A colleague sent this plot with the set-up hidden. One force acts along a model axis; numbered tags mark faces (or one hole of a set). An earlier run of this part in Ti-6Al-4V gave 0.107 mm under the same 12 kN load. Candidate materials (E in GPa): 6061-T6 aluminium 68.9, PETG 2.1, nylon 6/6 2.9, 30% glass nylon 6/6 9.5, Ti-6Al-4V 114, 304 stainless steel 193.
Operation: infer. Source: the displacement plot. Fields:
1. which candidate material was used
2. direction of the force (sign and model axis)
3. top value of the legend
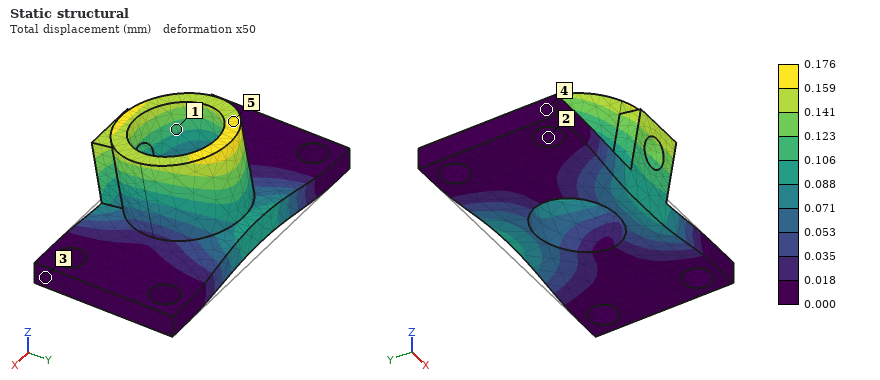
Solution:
6061-T6 aluminium
-Y
0.176 mm
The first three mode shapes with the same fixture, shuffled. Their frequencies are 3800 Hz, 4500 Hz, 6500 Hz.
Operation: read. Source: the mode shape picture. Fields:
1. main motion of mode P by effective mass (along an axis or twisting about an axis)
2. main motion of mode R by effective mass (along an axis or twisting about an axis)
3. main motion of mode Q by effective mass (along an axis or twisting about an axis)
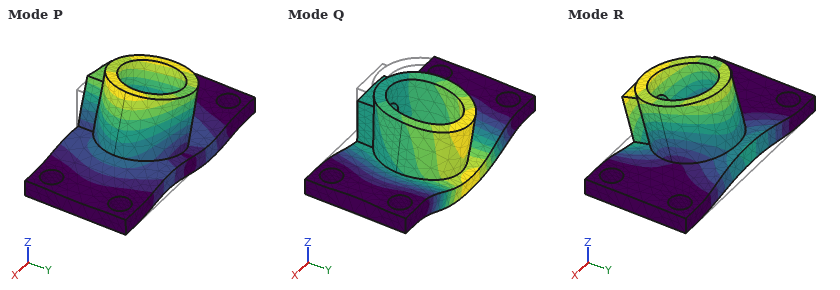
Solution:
along X
along Y
along Z
